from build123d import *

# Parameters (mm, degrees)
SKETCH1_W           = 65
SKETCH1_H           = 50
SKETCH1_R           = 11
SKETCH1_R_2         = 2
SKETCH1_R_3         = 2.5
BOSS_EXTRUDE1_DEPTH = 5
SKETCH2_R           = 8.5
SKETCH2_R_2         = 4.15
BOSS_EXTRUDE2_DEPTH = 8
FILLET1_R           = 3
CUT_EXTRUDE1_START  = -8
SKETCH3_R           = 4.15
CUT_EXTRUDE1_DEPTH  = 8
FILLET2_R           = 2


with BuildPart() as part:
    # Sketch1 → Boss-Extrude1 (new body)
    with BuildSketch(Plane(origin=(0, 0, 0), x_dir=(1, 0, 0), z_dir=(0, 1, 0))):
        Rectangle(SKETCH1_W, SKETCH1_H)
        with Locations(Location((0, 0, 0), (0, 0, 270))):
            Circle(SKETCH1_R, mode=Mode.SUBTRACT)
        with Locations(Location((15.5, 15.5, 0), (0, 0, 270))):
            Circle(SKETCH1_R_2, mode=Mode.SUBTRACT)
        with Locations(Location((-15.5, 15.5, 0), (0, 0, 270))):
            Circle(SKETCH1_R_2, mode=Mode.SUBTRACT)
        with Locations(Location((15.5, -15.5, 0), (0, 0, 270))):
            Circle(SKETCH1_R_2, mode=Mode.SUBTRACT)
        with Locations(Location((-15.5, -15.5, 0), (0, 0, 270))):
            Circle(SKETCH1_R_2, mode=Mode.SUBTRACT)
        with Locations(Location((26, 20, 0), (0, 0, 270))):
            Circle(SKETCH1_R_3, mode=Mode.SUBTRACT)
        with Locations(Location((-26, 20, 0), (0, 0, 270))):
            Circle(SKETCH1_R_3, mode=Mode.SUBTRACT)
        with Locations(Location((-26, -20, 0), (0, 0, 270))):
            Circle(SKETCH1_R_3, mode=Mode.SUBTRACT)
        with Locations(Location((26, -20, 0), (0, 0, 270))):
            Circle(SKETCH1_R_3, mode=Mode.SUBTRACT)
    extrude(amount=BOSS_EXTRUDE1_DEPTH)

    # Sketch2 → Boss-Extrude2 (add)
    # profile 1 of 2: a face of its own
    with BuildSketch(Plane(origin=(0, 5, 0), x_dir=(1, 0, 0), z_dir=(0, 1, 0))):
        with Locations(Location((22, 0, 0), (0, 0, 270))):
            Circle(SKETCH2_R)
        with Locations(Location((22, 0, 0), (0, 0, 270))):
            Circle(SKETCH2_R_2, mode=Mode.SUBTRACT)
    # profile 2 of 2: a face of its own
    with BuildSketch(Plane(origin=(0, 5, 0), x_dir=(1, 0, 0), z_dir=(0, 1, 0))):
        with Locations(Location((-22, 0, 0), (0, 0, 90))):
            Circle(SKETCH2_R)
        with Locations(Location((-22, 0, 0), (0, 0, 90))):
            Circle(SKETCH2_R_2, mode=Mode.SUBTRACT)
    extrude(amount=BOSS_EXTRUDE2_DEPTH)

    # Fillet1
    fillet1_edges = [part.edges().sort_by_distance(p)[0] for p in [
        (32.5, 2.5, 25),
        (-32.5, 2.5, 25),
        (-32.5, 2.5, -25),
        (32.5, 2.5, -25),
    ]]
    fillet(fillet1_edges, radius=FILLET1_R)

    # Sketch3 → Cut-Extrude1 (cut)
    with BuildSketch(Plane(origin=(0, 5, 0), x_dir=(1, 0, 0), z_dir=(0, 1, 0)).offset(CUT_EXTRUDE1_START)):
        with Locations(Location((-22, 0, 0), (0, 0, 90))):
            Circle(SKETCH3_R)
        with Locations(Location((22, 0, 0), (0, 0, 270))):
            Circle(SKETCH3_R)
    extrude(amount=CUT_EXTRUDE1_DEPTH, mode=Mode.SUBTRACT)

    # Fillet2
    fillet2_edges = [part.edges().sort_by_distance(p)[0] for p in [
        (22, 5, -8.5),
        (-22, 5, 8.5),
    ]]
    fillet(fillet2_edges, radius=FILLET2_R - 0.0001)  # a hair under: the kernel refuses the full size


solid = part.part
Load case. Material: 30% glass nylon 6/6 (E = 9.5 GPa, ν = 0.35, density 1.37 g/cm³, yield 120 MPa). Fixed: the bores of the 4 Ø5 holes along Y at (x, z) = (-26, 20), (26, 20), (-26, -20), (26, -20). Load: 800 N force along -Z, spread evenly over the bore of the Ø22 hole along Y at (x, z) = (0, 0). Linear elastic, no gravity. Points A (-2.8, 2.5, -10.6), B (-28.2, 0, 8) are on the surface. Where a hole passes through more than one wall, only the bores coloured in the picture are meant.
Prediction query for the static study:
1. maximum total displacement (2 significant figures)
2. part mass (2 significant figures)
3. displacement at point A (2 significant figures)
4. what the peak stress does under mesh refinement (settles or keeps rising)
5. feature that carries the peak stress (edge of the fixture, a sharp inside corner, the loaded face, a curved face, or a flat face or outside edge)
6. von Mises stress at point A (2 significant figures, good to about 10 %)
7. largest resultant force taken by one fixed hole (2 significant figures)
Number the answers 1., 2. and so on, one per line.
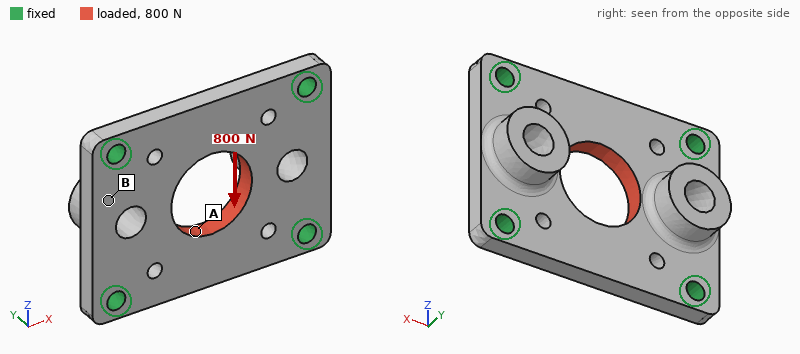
1. 17 µm
2. 22 g
3. 16 µm
4. keeps rising
5. edge of the fixture
6. 2.4 MPa
7. 230 N
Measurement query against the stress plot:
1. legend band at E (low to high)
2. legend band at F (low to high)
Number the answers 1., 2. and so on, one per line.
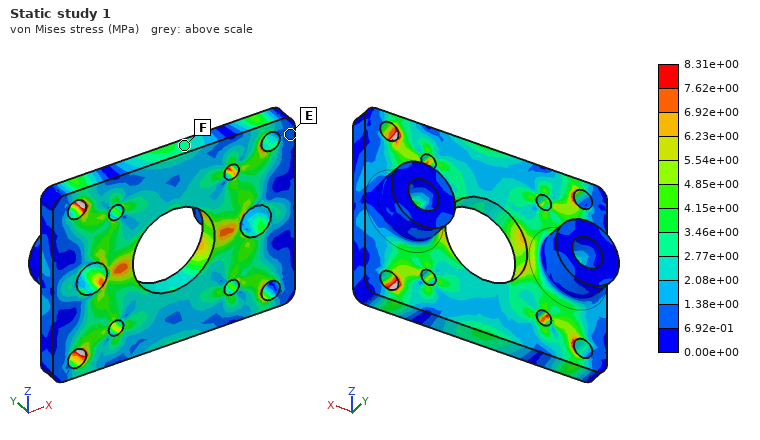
1. 6.92e-01 to 1.38e+00 MPa
2. 2.77e+00 to 3.46e+00 MPa
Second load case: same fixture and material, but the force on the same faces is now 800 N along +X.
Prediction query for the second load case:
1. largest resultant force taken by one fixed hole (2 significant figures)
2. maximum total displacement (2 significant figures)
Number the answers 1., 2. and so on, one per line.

1. 210 N
2. 9.5 µm
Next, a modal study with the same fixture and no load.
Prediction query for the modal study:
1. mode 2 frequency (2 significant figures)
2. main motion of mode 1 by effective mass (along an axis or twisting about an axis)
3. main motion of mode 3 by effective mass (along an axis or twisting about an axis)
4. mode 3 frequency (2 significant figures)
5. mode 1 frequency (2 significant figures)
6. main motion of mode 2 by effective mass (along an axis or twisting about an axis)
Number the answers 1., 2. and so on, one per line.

1. 6100 Hz
2. along Y
3. twisting about Z
4. 7400 Hz
5. 4300 Hz
6. twisting about X
